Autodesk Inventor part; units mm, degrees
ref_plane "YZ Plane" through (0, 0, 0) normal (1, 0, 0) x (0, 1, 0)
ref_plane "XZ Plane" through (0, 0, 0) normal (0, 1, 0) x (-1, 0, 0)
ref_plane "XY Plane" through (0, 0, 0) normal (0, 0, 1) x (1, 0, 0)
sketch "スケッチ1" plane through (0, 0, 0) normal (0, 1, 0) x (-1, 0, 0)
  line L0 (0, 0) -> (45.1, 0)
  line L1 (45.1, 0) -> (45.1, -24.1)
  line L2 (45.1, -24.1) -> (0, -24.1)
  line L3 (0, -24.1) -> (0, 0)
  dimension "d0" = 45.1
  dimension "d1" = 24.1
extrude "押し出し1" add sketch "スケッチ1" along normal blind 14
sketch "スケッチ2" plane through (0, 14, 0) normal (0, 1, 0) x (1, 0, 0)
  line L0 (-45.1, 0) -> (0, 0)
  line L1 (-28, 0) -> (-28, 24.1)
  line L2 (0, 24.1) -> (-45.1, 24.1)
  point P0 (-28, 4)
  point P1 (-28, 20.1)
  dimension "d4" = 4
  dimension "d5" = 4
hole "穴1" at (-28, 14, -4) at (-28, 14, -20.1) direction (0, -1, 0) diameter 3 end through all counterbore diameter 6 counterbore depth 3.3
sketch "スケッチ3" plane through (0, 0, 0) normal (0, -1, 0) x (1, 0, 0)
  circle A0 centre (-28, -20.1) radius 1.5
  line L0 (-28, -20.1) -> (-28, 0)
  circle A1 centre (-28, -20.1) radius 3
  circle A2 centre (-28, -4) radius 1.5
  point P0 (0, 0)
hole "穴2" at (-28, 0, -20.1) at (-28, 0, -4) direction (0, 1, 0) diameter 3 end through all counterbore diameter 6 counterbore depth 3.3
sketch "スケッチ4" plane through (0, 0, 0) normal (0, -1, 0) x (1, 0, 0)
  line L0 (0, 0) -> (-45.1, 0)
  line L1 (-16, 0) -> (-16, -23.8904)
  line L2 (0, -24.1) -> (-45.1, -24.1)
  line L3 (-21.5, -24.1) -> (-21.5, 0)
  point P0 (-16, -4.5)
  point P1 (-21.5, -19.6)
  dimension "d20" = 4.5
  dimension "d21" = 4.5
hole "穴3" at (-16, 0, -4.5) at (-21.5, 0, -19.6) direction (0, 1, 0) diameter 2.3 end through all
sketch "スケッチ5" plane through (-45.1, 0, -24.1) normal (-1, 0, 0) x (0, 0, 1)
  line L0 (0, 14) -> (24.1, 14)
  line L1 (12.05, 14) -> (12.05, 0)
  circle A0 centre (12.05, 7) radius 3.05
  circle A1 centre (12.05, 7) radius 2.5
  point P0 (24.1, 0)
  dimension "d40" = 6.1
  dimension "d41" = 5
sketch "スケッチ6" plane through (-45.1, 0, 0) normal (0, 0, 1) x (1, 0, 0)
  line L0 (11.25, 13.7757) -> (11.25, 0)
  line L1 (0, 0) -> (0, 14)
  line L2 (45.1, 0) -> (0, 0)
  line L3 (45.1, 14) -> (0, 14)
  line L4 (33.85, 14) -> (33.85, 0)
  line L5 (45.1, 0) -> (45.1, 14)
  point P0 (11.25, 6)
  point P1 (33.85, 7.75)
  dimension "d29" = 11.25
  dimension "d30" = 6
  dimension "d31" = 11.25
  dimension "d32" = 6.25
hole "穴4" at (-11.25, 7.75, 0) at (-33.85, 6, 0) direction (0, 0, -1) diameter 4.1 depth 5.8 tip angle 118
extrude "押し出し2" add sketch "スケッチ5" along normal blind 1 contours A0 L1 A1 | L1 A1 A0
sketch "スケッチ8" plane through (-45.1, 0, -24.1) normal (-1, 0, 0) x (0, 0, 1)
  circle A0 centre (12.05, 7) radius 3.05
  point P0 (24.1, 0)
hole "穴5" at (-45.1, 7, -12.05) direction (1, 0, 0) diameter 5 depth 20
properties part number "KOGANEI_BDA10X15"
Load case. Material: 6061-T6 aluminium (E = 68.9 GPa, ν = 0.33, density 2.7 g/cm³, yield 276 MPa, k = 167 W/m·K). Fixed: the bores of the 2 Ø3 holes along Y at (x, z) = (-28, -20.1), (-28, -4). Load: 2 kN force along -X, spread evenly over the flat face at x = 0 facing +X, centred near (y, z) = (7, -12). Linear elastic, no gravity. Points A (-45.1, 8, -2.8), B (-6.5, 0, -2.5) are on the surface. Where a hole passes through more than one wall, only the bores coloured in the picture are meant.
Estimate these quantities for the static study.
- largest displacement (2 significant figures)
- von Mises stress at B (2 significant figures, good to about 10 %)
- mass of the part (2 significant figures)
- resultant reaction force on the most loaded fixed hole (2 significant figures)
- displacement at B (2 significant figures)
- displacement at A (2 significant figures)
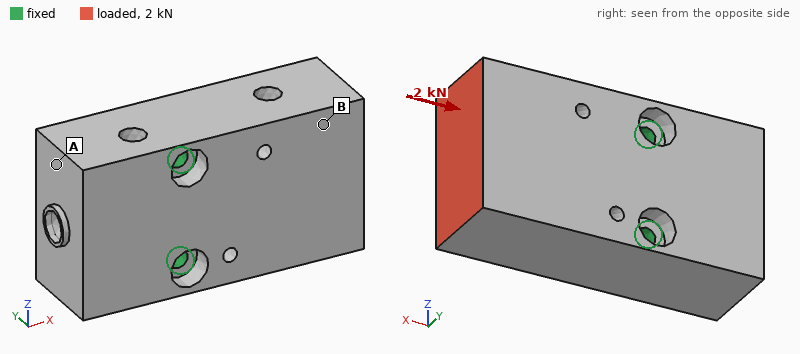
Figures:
3.3 µm
6.5 MPa
38 g
1.0 kN
2.6 µm
0.51 µm
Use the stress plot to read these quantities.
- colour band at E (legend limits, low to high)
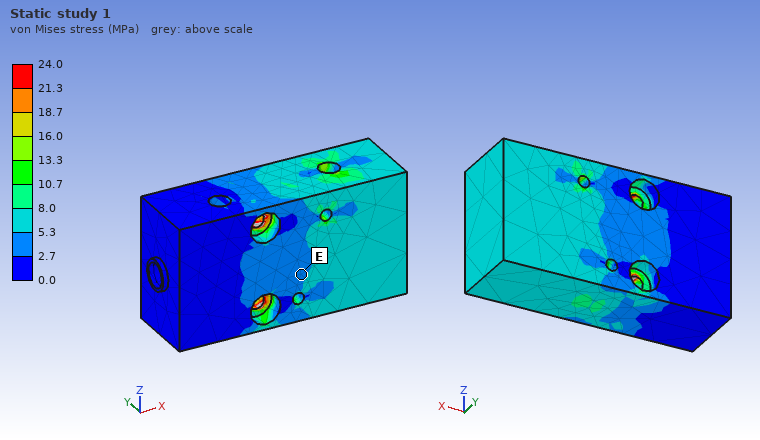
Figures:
2.7 to 5.3 MPa
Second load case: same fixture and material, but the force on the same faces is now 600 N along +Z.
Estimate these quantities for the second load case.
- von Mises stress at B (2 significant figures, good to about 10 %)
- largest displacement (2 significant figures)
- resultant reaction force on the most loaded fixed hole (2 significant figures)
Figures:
3.2 MPa
9.2 µm
1.0 kN
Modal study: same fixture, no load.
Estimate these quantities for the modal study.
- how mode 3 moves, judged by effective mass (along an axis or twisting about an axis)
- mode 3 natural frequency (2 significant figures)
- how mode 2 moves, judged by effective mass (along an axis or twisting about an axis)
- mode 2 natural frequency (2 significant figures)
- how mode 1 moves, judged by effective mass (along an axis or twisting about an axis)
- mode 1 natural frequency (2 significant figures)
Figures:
along Y
19 kHz
along Z
15 kHz
along Y
7000 Hz
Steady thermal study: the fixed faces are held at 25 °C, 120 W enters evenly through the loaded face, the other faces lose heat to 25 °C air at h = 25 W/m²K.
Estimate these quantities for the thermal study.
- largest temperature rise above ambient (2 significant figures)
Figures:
69 K
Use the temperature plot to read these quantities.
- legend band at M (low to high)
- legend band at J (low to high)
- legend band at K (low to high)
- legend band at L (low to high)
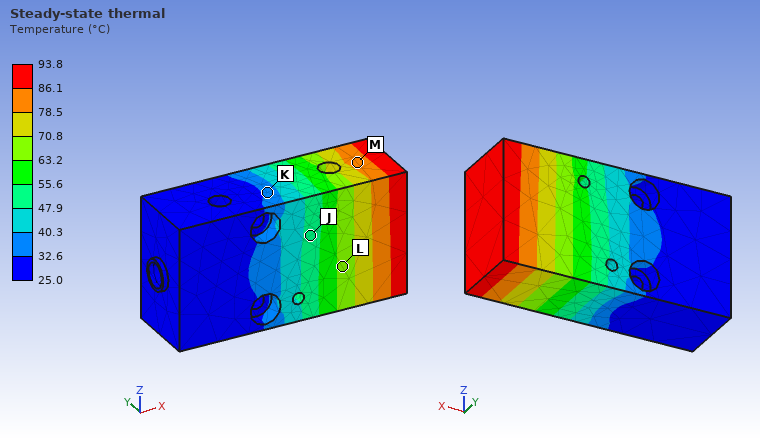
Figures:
78.5 to 86.1 °C
47.9 to 55.6 °C
32.6 to 40.3 °C
63.2 to 70.8 °C
